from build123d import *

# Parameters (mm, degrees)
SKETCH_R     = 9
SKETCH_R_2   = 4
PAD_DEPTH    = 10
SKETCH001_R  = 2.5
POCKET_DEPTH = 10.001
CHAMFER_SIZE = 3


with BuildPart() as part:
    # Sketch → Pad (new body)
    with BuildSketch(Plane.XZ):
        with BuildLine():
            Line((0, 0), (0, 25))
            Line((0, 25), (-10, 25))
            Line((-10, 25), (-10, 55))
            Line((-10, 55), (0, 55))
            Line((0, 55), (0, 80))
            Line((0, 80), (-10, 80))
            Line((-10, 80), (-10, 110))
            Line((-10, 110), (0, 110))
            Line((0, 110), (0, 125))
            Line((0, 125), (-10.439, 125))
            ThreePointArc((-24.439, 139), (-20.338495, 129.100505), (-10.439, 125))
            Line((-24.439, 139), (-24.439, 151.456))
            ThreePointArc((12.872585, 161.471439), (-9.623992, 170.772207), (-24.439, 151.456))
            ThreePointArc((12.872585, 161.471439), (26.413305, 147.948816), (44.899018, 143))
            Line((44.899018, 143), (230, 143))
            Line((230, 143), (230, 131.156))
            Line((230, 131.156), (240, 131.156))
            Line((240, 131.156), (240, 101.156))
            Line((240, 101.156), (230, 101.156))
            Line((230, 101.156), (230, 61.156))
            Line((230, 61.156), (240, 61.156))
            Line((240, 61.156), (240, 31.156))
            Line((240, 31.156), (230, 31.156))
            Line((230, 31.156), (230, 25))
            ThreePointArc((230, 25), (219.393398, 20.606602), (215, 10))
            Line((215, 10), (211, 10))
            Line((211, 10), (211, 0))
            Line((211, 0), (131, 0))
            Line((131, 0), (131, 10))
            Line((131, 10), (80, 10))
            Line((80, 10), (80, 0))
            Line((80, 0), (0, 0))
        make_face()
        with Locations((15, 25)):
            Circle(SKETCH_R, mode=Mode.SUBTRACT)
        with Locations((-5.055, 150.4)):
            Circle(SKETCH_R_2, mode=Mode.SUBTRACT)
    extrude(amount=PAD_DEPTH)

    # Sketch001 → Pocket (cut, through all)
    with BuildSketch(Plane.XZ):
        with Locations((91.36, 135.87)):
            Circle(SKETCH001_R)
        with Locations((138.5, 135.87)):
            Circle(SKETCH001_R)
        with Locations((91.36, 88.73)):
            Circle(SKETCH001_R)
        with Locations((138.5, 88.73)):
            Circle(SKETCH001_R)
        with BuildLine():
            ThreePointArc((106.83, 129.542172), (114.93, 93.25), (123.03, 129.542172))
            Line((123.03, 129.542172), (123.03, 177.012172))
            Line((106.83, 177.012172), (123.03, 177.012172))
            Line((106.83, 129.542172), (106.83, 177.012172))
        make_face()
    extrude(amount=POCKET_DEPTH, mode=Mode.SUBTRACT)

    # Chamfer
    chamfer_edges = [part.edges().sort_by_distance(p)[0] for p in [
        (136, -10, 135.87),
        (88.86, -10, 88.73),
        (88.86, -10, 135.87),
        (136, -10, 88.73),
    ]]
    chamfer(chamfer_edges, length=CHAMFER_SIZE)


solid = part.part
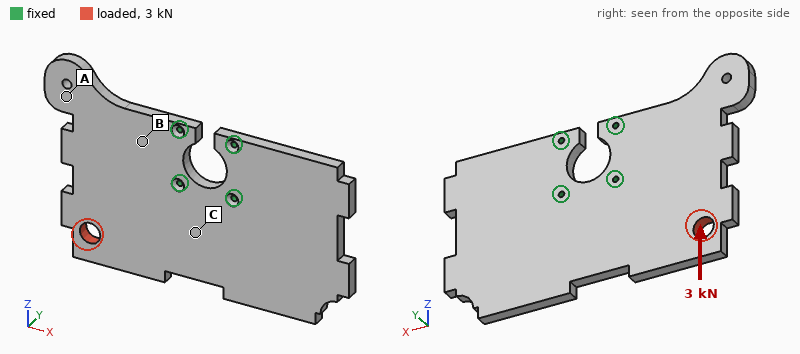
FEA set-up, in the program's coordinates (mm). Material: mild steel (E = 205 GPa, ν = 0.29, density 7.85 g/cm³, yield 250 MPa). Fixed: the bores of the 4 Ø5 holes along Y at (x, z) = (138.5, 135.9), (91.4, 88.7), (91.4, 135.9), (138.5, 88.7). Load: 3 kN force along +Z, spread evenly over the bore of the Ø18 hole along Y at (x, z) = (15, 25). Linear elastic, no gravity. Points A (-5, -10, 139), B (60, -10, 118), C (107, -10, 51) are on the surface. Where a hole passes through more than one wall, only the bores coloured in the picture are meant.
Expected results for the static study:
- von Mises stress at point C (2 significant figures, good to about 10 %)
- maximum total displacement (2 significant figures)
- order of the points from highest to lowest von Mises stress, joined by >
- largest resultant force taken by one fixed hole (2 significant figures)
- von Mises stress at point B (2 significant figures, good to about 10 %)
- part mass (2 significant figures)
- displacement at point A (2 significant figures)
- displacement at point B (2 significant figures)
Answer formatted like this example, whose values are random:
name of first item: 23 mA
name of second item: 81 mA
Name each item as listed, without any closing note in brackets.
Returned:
von Mises stress at point C: 3.8 MPa
maximum total displacement: 13 µm
order of the points from highest to lowest von Mises stress, joined by >: B > C > A
largest resultant force taken by one fixed hole: 3.3 kN
von Mises stress at point B: 7.5 MPa
part mass: 2.6 kg
displacement at point A: 9.0 µm
displacement at point B: 3.1 µm
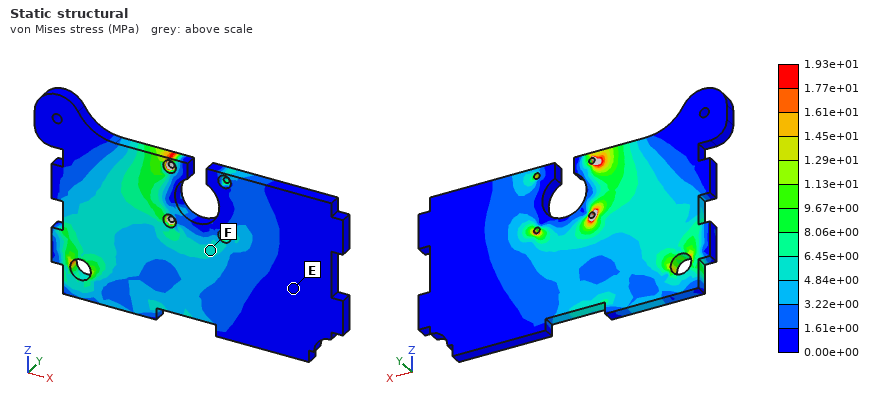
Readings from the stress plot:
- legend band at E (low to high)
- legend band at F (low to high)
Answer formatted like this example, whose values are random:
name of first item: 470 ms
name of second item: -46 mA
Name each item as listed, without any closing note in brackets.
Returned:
legend band at E: 0.00e+00 to 1.61e+00 MPa
legend band at F: 4.84e+00 to 6.45e+00 MPa
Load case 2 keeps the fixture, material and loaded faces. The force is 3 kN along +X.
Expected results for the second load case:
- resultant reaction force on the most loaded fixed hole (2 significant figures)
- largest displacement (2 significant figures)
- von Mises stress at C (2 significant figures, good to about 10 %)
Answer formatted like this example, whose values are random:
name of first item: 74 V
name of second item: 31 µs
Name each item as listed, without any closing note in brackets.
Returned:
resultant reaction force on the most loaded fixed hole: 2.9 kN
largest displacement: 11 µm
von Mises stress at C: 5.6 MPa
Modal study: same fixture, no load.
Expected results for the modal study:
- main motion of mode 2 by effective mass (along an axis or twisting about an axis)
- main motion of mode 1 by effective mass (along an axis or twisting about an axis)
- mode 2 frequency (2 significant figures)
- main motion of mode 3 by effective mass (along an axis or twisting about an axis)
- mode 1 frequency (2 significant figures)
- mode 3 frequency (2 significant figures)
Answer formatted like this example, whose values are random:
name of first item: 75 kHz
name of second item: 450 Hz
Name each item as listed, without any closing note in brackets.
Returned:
main motion of mode 2 by effective mass: along Y
main motion of mode 1 by effective mass: along Y
mode 2 frequency: 650 Hz
main motion of mode 3 by effective mass: twisting about X
mode 1 frequency: 560 Hz
mode 3 frequency: 750 Hz
